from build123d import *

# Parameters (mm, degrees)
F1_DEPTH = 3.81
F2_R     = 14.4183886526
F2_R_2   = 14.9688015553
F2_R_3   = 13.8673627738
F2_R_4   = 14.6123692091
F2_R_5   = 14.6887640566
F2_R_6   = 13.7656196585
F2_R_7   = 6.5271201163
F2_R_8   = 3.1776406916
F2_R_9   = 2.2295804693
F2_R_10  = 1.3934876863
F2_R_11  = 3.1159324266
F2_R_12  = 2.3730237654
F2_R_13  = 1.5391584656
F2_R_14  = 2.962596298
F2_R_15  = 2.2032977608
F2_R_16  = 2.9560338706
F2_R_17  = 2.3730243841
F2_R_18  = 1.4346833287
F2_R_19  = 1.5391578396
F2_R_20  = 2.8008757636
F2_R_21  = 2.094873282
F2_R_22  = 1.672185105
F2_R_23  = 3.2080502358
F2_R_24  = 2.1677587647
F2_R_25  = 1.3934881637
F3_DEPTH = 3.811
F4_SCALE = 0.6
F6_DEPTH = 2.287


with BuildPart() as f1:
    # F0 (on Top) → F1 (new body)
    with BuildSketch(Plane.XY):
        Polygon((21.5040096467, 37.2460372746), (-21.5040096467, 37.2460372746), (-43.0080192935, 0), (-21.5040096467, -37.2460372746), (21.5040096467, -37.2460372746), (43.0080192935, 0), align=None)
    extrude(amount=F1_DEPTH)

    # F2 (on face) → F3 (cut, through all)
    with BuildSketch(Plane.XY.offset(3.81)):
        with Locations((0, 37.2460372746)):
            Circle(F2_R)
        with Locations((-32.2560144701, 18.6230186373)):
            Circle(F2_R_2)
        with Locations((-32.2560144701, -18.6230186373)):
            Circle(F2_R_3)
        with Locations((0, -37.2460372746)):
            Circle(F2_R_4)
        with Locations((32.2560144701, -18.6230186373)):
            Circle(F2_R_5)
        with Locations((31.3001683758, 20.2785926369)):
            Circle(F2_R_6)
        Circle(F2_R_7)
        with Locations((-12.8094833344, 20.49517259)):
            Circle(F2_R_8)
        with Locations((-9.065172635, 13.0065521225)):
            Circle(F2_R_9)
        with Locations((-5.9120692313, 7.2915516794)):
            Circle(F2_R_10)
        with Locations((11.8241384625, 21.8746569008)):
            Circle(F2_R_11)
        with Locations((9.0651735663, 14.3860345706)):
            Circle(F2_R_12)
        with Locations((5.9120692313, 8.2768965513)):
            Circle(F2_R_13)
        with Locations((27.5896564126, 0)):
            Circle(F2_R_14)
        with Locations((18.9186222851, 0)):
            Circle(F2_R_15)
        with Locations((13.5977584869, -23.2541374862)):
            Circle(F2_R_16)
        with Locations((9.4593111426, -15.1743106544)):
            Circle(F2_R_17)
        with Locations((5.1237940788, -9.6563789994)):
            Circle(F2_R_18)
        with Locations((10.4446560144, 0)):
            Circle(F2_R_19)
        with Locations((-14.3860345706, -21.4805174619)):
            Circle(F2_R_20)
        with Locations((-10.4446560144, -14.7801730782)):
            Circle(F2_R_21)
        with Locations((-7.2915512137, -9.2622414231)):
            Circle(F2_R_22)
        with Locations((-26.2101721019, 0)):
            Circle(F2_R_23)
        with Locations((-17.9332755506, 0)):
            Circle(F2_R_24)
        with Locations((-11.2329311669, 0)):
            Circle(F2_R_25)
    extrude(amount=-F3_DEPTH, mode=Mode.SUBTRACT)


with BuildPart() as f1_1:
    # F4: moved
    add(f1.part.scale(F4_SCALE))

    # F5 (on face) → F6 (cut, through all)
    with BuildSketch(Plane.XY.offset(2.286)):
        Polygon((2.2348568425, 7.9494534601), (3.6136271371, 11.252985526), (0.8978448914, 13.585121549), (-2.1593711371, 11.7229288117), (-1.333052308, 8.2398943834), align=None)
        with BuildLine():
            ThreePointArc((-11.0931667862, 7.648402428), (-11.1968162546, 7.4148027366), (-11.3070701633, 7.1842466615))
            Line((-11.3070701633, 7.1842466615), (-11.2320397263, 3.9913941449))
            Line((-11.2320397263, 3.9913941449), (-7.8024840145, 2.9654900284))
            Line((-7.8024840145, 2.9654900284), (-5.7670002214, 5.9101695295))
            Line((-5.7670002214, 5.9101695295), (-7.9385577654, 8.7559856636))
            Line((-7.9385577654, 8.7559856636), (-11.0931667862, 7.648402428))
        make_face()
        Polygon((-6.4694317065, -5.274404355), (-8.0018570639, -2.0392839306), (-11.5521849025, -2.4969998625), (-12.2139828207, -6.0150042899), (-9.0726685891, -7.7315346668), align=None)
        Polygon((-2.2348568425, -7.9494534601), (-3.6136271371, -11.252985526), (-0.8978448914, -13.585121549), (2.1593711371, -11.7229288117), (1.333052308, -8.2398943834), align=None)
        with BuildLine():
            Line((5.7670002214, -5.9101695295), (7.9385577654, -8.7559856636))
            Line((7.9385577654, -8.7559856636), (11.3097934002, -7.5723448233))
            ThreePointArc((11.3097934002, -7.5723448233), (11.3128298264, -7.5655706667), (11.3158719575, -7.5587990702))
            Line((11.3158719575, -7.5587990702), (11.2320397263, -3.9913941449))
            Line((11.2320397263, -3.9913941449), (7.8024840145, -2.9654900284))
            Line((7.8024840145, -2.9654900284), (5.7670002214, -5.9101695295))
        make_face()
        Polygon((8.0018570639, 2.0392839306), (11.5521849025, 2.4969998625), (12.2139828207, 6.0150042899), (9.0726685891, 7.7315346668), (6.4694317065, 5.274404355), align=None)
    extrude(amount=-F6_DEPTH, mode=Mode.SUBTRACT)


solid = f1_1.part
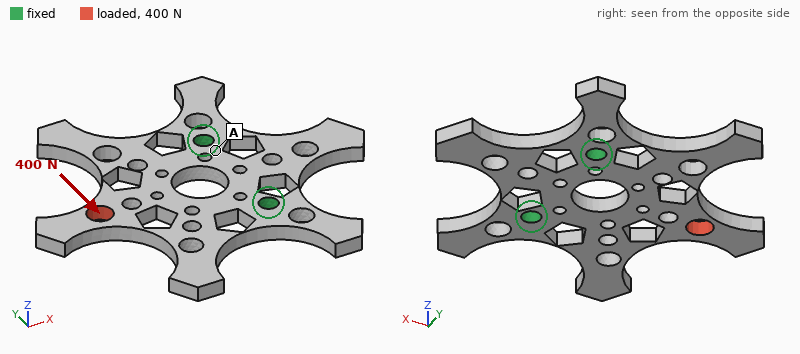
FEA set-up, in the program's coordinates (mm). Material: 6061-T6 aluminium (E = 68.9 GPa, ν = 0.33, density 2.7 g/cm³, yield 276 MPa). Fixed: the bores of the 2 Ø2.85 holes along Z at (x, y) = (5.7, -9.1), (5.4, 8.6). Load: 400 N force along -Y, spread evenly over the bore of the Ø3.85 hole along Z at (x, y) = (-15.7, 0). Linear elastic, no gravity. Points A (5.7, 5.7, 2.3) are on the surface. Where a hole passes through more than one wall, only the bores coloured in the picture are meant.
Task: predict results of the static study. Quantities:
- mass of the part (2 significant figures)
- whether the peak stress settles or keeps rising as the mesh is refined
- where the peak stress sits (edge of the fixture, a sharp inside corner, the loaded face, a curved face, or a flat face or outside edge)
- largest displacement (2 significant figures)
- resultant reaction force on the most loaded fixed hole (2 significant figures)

4.5 g
keeps rising
a sharp inside corner
91 µm
500 N
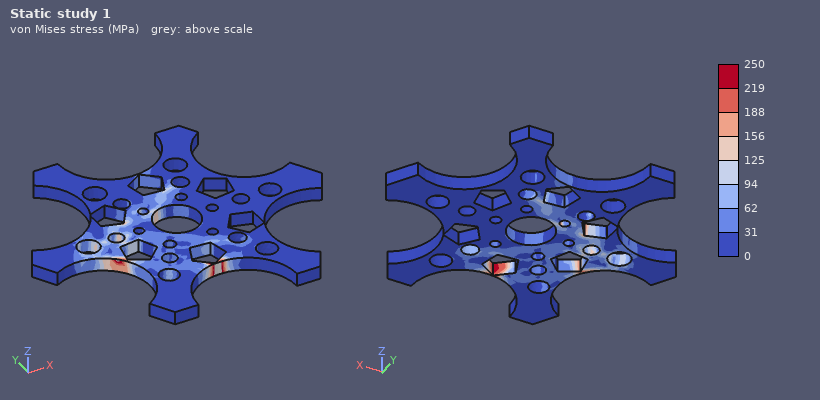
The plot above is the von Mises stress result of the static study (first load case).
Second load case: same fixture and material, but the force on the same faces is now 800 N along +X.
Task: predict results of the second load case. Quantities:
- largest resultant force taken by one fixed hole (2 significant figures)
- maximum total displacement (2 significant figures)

460 N
34 µm
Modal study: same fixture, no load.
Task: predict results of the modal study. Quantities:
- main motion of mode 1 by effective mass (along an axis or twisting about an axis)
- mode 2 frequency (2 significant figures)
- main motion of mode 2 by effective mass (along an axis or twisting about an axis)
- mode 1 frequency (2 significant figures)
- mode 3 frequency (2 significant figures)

along Z
3600 Hz
twisting about X
2300 Hz
4200 Hz
